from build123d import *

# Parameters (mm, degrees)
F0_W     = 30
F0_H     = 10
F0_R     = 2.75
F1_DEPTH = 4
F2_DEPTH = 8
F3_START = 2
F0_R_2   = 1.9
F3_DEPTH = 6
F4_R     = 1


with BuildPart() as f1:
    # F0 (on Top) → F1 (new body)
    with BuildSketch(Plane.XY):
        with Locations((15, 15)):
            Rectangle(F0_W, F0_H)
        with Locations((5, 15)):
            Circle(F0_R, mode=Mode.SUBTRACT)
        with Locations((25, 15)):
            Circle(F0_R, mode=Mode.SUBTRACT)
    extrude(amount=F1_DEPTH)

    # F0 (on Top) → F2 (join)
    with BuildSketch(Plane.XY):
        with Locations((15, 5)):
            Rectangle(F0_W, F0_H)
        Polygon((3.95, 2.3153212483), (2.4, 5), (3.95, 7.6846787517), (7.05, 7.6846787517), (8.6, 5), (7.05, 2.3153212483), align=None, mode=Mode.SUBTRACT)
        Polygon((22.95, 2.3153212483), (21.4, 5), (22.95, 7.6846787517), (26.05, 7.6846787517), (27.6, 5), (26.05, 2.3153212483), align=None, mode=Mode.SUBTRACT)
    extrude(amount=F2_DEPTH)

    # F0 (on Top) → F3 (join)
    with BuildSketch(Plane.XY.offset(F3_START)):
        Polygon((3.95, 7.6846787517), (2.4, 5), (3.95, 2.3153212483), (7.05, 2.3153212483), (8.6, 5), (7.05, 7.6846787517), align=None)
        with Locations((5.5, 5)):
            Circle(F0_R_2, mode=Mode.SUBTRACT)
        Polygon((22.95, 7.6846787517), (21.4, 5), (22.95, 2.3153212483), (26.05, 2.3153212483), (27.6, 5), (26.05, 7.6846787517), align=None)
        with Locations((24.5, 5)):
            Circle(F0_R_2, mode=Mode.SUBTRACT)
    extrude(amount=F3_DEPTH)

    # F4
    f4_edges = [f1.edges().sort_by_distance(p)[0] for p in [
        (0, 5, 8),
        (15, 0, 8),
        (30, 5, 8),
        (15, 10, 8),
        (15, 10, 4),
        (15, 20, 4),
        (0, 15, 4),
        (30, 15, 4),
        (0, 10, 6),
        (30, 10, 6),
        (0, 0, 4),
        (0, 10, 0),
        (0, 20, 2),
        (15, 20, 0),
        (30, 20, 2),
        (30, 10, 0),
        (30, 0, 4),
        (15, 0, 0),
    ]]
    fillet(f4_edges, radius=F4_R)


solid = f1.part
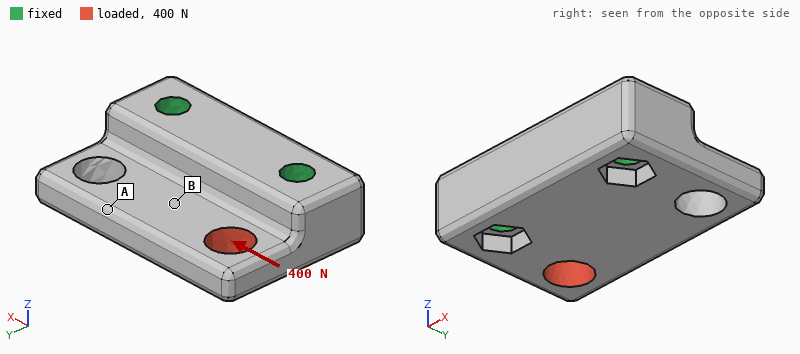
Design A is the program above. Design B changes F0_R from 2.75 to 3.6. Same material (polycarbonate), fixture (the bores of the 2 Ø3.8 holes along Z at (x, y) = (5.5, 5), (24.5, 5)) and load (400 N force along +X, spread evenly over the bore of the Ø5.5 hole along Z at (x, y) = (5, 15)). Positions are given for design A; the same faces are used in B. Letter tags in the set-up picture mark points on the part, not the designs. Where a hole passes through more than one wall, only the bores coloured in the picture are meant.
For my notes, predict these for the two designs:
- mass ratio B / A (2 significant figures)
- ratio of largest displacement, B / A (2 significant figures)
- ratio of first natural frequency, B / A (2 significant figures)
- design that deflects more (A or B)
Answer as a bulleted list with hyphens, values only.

- 0.96
- 1.6
- 0.99
- B
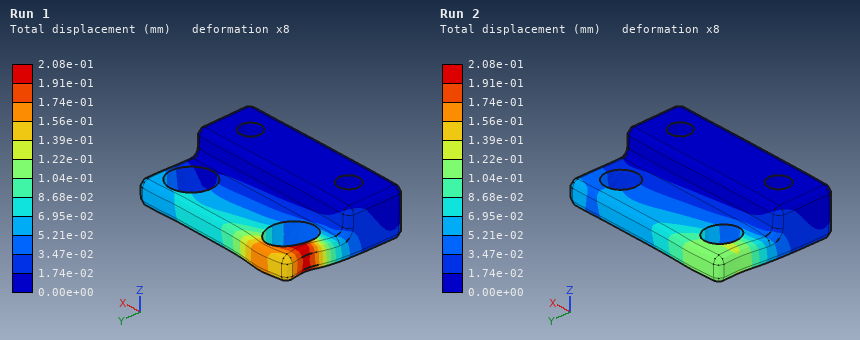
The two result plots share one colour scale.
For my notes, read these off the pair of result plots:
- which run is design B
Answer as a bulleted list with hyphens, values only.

- Run 1
